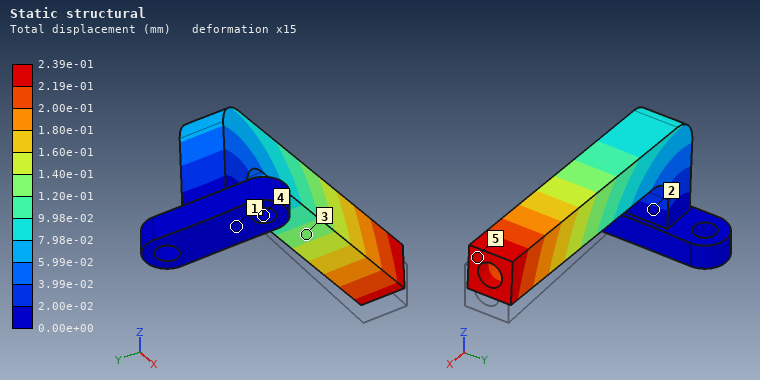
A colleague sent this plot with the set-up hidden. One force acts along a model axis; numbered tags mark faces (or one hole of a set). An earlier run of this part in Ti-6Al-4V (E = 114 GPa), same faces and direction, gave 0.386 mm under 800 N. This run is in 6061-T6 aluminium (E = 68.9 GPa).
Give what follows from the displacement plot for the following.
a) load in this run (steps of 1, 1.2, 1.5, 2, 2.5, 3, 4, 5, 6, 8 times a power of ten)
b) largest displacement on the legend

300 N
2.39e-01 mm
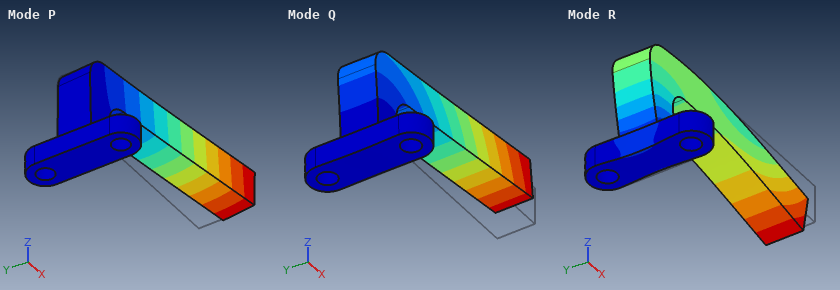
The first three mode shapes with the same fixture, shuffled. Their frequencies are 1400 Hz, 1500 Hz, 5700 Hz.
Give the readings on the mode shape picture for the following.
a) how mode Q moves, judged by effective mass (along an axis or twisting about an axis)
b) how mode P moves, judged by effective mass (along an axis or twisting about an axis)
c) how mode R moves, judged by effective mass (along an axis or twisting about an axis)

along Z
along Y
along X
